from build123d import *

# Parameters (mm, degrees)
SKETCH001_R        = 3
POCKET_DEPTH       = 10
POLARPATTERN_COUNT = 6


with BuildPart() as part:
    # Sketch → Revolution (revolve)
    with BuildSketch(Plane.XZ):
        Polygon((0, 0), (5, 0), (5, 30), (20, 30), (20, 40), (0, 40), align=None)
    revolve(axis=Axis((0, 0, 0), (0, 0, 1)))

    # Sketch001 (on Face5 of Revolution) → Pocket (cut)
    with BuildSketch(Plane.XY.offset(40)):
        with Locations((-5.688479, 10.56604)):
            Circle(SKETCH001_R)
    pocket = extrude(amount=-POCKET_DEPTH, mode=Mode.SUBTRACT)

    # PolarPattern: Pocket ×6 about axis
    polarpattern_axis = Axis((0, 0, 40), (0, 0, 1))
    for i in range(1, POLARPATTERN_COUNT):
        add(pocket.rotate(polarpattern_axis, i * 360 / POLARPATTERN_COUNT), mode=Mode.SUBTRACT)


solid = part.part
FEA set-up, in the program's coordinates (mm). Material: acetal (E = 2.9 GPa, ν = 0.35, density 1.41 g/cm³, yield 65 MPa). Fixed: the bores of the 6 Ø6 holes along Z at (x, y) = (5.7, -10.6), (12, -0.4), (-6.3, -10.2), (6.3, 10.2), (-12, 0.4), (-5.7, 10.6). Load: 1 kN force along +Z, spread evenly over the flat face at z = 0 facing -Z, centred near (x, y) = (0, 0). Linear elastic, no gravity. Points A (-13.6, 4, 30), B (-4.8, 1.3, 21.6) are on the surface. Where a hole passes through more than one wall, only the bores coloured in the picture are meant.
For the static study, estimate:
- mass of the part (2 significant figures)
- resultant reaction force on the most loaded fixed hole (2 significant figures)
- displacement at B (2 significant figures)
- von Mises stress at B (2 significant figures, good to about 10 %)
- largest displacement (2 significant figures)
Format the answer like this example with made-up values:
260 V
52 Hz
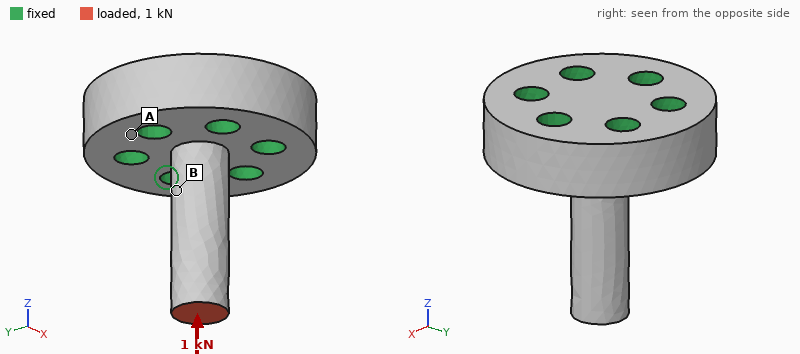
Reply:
19 g
200 N
0.058 mm
13 MPa
0.15 mm
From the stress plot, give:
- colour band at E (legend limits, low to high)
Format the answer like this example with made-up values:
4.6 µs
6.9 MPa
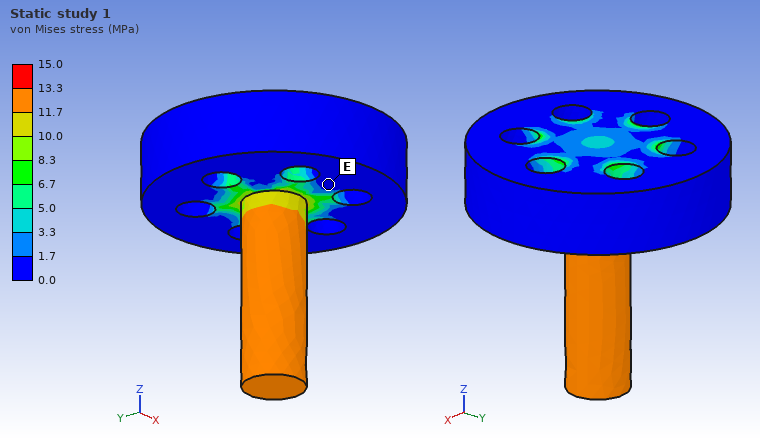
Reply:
0.0 to 1.7 MPa
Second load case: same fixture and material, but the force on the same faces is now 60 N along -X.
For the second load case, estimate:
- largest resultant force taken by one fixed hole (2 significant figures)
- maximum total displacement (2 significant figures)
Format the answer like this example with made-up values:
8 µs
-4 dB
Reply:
76 N
0.49 mm
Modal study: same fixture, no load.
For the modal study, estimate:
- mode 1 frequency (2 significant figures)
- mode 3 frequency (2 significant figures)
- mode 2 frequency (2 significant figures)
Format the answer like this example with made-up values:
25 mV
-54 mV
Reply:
1900 Hz
6900 Hz
1900 Hz
